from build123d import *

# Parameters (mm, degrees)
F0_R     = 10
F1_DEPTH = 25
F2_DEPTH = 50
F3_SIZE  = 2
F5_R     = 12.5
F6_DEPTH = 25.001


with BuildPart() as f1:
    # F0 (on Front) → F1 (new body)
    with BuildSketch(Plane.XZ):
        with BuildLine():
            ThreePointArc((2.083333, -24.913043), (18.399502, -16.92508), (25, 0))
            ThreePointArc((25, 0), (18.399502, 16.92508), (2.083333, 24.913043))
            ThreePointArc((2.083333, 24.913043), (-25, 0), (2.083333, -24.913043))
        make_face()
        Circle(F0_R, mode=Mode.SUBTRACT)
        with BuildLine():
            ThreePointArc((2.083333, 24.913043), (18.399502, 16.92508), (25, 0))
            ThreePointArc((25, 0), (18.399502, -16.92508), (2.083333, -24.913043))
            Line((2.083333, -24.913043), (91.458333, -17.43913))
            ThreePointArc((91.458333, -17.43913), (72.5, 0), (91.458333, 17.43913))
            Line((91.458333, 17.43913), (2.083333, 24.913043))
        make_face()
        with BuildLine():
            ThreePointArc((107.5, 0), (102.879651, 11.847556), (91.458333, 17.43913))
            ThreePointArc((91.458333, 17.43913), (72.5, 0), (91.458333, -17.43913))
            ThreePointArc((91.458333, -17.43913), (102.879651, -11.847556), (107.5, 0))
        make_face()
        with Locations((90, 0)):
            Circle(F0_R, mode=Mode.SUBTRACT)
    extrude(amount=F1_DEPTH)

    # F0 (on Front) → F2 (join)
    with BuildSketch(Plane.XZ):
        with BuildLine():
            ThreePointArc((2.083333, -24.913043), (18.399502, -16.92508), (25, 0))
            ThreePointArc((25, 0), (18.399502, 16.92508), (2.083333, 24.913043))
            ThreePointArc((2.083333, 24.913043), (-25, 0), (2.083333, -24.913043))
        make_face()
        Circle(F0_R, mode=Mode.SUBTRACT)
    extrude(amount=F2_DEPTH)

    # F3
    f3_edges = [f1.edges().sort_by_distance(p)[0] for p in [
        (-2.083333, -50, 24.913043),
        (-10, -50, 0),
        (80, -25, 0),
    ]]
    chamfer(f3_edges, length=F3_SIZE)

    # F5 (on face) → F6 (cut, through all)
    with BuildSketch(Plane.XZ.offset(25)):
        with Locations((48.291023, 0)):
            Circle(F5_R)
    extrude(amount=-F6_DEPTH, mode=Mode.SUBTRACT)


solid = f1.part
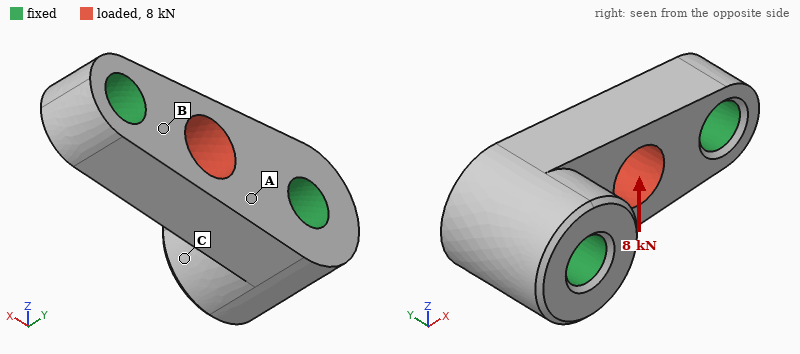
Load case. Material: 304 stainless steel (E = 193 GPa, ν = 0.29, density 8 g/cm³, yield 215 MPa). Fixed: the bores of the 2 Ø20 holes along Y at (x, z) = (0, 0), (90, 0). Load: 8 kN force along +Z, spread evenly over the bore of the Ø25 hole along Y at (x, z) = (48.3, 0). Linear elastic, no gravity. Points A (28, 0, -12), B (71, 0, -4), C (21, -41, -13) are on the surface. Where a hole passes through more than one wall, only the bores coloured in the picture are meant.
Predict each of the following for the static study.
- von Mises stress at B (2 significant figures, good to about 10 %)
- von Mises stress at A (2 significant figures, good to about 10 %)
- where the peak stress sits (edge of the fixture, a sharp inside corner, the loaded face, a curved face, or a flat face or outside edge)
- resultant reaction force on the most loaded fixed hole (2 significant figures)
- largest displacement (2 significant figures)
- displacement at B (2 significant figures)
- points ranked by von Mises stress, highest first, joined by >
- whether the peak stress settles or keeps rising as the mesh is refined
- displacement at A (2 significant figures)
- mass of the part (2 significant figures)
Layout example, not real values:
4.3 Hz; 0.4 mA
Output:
12 MPa; 6.4 MPa; edge of the fixture; 4.1 kN; 3.2 µm; 1.1 µm; B > A > C; keeps rising; 1.6 µm; 1.2 kg
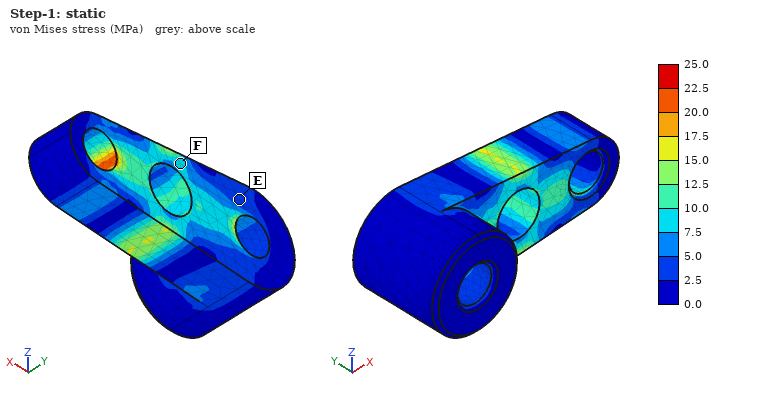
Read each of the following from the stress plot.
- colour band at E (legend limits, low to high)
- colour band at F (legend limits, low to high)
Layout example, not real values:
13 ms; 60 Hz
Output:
2.5 to 5.0 MPa; 7.5 to 10.0 MPa
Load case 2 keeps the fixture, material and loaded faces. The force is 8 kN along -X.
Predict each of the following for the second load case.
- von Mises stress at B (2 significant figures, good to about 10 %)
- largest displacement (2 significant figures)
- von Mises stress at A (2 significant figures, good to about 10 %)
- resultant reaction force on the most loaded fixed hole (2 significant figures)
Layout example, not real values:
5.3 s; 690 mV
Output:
4.9 MPa; 0.87 µm; 3.7 MPa; 4.1 kN
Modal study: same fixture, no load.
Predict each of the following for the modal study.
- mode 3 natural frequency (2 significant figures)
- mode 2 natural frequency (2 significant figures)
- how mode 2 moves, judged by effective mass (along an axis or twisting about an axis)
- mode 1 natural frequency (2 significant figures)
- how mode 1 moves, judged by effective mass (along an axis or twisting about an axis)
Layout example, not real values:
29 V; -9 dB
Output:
18 kHz; 17 kHz; along Z; 16 kHz; along Y
